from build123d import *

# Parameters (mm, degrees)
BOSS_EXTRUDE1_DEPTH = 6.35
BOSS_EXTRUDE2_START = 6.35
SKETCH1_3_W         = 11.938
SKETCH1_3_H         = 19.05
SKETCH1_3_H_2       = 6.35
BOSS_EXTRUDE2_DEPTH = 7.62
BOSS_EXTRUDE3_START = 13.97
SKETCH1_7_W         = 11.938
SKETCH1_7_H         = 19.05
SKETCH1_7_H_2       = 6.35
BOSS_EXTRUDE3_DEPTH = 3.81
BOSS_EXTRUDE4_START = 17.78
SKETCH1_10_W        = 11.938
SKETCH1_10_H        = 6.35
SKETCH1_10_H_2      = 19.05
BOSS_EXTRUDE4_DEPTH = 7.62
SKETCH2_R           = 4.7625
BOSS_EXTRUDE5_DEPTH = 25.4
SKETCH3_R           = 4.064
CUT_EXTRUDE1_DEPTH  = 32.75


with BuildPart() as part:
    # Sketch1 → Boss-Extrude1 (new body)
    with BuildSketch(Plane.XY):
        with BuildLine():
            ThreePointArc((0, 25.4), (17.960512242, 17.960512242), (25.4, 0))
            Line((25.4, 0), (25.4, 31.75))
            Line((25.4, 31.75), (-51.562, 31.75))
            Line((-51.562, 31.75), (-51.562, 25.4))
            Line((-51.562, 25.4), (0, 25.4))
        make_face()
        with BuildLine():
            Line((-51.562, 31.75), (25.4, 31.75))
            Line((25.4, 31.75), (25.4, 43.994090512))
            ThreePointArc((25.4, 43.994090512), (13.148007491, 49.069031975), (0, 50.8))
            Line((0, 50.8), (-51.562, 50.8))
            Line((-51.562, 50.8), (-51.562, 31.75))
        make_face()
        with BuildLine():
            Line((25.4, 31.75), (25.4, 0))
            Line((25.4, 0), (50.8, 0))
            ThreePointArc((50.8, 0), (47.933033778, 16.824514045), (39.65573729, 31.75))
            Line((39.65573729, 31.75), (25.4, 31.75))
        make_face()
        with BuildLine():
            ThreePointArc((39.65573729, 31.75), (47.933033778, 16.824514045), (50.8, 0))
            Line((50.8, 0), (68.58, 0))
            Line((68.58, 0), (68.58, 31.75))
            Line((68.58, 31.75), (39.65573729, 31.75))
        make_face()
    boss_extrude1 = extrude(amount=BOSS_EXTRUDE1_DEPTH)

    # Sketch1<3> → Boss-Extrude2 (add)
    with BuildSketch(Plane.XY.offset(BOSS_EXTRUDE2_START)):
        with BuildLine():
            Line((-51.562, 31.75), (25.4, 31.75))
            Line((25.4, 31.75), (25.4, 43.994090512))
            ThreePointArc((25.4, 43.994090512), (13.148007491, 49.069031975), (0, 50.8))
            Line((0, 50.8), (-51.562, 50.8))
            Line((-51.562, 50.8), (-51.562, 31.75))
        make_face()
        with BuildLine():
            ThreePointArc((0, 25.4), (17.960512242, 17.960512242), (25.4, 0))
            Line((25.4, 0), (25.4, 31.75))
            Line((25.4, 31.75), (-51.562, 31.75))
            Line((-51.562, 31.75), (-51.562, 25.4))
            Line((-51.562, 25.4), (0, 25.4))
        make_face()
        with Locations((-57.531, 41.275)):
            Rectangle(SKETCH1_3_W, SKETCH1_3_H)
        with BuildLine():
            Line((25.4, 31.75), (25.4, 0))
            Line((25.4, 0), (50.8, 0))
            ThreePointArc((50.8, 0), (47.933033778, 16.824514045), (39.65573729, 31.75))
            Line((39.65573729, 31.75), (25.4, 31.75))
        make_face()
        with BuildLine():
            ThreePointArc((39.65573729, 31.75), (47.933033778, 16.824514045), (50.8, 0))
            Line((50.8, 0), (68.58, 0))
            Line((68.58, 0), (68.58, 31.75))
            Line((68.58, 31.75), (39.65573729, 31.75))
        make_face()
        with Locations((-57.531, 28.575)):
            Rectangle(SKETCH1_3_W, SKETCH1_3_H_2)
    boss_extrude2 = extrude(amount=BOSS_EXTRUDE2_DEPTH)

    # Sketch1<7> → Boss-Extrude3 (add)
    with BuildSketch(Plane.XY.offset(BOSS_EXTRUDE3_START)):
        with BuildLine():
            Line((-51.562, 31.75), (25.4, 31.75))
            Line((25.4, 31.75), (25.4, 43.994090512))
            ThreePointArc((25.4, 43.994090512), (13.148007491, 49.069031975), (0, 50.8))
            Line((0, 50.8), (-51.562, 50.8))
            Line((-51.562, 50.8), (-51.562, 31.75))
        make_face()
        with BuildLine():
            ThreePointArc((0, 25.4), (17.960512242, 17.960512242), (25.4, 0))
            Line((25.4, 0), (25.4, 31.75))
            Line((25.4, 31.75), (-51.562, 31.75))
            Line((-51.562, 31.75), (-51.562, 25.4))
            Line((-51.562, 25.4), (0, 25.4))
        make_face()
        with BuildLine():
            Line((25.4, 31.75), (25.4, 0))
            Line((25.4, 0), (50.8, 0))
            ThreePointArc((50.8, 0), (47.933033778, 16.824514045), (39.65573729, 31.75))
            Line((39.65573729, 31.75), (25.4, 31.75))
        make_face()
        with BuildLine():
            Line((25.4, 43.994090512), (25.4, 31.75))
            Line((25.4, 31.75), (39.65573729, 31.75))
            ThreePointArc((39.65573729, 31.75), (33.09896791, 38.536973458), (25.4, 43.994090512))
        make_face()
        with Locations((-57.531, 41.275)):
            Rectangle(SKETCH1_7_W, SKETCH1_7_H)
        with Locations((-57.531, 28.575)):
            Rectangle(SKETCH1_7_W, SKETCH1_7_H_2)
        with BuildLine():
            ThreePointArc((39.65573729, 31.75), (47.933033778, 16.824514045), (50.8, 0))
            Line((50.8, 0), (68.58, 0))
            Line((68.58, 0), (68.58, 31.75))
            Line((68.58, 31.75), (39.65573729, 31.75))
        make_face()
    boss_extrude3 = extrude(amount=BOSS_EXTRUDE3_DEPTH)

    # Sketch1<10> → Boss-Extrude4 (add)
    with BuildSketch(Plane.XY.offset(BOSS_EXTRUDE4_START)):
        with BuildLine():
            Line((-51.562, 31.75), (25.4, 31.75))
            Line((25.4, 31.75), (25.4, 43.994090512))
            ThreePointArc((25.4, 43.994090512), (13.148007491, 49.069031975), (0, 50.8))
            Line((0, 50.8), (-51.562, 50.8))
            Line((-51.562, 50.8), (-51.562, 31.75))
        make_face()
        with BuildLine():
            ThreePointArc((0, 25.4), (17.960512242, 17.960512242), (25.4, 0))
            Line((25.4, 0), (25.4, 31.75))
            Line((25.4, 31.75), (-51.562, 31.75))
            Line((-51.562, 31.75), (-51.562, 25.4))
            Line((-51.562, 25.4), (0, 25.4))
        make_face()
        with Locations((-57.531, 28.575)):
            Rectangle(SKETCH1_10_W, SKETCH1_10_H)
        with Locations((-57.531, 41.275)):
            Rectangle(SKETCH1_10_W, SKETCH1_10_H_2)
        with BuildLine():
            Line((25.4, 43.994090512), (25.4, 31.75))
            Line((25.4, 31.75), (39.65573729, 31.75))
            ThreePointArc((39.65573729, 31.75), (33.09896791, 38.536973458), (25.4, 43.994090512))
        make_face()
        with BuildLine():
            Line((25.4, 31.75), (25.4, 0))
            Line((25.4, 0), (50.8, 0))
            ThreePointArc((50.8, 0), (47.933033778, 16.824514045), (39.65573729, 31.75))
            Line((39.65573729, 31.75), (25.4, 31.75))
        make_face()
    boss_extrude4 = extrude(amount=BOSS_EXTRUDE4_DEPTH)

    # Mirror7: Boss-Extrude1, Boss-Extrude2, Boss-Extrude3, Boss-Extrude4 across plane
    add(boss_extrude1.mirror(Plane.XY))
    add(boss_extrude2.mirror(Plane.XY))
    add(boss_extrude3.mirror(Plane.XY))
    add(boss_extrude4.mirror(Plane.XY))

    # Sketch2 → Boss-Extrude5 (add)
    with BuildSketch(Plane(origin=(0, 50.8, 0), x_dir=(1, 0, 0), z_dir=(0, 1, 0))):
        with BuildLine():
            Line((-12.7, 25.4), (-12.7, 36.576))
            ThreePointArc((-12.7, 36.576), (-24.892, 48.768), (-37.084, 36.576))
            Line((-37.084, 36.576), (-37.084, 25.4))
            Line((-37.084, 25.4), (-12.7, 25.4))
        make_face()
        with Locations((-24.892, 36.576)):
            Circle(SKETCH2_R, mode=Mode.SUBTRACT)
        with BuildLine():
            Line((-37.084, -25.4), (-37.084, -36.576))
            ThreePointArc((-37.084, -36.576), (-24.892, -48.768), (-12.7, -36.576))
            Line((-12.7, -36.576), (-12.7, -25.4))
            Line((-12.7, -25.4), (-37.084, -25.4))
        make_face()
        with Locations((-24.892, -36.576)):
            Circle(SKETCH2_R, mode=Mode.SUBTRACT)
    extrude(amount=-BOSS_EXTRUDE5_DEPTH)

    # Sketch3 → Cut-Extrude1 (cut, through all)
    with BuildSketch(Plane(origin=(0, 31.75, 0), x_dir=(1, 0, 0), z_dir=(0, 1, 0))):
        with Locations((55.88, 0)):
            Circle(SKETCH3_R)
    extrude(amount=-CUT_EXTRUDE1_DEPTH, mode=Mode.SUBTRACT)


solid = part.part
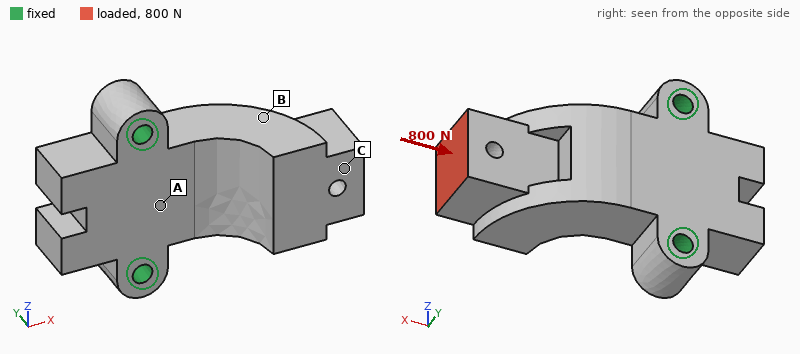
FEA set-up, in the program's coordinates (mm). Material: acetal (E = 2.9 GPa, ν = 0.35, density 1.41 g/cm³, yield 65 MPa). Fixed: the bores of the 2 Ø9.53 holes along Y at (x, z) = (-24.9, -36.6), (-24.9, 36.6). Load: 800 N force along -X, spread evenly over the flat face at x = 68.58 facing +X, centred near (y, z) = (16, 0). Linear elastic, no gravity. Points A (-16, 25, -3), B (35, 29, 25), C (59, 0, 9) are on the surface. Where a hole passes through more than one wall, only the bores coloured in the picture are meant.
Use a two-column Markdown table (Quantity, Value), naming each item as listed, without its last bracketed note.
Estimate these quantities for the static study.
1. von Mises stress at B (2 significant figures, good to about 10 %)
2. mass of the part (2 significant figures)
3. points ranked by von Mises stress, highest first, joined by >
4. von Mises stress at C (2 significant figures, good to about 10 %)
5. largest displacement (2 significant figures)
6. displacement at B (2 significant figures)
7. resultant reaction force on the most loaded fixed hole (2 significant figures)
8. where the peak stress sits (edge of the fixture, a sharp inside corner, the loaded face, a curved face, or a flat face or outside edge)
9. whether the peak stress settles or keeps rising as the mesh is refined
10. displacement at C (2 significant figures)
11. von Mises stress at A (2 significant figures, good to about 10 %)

| Quantity | Value |
|---|---|
| von Mises stress at B | 1.2 MPa |
| mass of the part | 280 g |
| points ranked by von Mises stress, highest first, joined by > | A > B > C |
| von Mises stress at C | 0.75 MPa |
| largest displacement | 0.55 mm |
| displacement at B | 0.26 mm |
| resultant reaction force on the most loaded fixed hole | 410 N |
| where the peak stress sits | edge of the fixture |
| whether the peak stress settles or keeps rising as the mesh is refined | keeps rising |
| displacement at C | 0.49 mm |
| von Mises stress at A | 2.3 MPa |
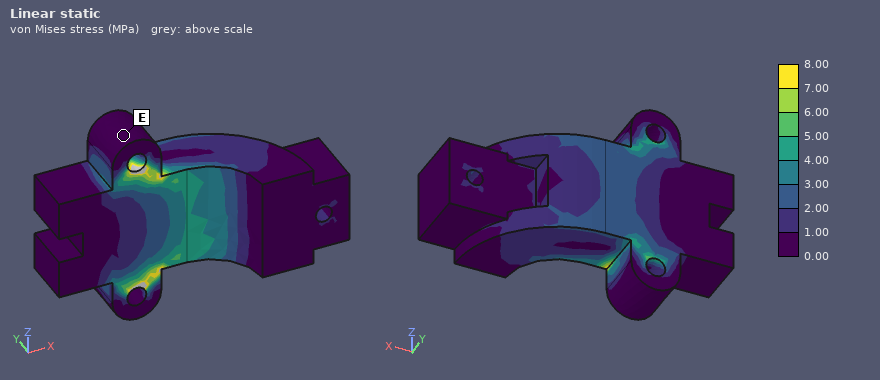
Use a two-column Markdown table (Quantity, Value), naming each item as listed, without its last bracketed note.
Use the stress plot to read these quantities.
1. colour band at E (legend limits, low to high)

| Quantity | Value |
|---|---|
| colour band at E | 0.00 to 1.00 MPa |
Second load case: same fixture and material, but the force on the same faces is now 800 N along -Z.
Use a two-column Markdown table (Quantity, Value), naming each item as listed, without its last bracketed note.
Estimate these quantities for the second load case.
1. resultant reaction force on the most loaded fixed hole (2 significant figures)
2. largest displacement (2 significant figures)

| Quantity | Value |
|---|---|
| resultant reaction force on the most loaded fixed hole | 1.2 kN |
| largest displacement | 0.47 mm |
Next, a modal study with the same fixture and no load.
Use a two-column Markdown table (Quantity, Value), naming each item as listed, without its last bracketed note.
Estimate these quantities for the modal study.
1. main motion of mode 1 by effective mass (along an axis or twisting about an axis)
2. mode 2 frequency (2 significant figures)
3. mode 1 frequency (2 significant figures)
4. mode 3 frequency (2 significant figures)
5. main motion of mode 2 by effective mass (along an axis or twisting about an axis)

| Quantity | Value |
|---|---|
| main motion of mode 1 by effective mass | along Y |
| mode 2 frequency | 960 Hz |
| mode 1 frequency | 450 Hz |
| mode 3 frequency | 1700 Hz |
| main motion of mode 2 by effective mass | along Z |
